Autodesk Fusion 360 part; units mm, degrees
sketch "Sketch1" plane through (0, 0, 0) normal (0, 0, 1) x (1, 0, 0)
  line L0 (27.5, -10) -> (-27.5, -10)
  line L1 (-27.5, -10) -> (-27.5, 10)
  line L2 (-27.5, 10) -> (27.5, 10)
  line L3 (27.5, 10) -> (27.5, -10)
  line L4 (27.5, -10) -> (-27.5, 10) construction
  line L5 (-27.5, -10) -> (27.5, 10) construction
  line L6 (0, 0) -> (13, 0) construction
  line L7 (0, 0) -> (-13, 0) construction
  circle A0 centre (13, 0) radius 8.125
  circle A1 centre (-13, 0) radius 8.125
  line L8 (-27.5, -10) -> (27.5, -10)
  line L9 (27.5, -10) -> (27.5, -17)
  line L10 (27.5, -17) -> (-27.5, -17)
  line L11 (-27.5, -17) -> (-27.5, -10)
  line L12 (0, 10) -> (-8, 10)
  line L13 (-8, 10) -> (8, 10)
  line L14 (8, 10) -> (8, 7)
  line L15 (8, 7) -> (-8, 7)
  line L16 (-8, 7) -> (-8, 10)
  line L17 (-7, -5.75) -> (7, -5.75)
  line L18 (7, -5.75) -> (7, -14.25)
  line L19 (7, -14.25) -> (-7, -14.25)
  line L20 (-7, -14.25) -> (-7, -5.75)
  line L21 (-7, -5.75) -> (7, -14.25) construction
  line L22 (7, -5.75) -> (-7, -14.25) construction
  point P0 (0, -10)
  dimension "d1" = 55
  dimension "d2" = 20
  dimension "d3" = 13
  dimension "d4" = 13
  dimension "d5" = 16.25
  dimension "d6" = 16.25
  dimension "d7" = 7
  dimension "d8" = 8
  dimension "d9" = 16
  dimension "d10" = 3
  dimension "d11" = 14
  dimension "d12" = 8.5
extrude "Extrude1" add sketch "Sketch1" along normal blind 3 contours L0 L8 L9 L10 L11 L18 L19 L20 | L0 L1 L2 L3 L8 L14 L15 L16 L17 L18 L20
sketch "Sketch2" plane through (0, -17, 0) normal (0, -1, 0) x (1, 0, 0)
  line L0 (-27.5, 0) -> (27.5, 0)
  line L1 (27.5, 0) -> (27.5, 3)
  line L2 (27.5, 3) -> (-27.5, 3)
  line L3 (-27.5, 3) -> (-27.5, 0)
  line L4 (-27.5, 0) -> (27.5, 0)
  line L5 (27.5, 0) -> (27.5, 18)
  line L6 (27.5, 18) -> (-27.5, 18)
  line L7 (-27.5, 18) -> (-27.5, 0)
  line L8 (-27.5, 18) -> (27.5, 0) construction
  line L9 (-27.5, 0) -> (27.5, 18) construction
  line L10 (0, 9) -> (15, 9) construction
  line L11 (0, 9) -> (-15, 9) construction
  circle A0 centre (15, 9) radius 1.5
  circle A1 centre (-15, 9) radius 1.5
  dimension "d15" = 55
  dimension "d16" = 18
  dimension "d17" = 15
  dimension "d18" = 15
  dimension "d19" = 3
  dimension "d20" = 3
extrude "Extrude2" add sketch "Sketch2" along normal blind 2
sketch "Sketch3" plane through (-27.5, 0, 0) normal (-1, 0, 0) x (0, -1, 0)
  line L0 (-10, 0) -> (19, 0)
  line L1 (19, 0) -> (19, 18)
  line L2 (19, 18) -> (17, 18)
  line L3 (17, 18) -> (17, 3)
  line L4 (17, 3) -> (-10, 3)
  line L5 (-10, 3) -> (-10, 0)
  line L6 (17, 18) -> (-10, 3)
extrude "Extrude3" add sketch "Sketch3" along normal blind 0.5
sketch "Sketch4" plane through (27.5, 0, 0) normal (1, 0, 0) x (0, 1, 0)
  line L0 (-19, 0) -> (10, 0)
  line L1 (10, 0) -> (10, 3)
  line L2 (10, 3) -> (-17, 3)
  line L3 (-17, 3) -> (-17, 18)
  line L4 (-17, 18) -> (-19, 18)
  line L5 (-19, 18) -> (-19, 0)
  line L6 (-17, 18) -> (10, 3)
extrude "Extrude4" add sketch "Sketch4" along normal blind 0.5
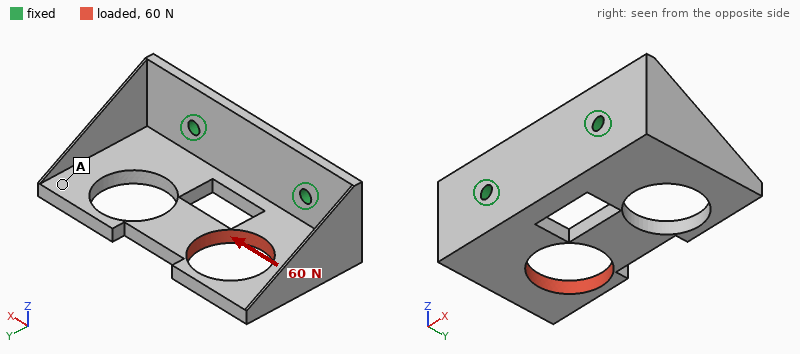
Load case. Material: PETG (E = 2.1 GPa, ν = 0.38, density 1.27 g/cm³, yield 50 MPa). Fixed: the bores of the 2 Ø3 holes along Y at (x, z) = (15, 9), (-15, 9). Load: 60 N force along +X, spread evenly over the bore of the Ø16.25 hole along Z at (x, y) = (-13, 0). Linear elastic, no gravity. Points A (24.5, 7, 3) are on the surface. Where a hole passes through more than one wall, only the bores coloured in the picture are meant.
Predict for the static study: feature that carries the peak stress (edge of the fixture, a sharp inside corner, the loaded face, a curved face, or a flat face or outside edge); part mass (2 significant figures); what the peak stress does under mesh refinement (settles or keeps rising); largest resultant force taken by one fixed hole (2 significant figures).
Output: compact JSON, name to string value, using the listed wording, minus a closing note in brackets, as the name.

{"feature that carries the peak stress": "a sharp inside corner", "part mass": "6.3 g", "what the peak stress does under mesh refinement": "keeps rising", "largest resultant force taken by one fixed hole": "47 N"}
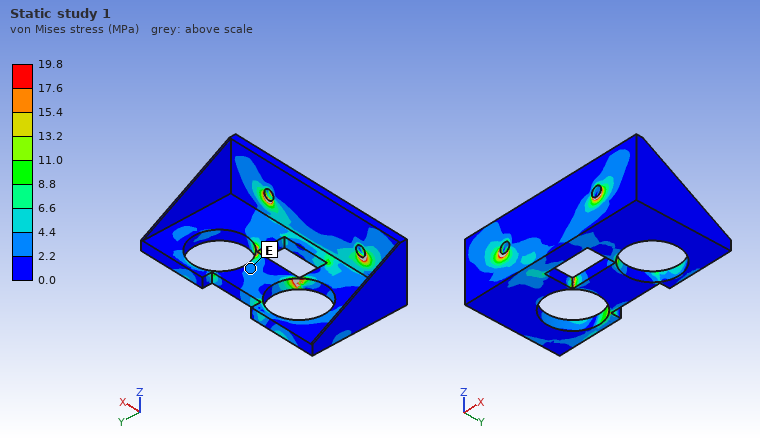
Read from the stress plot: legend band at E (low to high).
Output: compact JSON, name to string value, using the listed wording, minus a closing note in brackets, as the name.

{"legend band at E": "2.2 to 4.4 MPa"}
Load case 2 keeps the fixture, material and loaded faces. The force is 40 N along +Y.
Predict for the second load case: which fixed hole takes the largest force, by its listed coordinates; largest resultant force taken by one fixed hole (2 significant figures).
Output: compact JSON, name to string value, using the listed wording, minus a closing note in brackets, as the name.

{"which fixed hole takes the largest force, by its listed coordinates": "(-15, 9)", "largest resultant force taken by one fixed hole": "36 N"}
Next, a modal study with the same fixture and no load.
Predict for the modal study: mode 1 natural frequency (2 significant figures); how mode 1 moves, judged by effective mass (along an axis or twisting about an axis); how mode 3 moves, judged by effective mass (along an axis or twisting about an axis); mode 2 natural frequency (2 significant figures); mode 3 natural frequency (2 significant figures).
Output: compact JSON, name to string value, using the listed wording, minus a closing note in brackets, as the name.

{"mode 1 natural frequency": "510 Hz", "how mode 1 moves, judged by effective mass": "along Z", "how mode 3 moves, judged by effective mass": "along X", "mode 2 natural frequency": "700 Hz", "mode 3 natural frequency": "1500 Hz"}
